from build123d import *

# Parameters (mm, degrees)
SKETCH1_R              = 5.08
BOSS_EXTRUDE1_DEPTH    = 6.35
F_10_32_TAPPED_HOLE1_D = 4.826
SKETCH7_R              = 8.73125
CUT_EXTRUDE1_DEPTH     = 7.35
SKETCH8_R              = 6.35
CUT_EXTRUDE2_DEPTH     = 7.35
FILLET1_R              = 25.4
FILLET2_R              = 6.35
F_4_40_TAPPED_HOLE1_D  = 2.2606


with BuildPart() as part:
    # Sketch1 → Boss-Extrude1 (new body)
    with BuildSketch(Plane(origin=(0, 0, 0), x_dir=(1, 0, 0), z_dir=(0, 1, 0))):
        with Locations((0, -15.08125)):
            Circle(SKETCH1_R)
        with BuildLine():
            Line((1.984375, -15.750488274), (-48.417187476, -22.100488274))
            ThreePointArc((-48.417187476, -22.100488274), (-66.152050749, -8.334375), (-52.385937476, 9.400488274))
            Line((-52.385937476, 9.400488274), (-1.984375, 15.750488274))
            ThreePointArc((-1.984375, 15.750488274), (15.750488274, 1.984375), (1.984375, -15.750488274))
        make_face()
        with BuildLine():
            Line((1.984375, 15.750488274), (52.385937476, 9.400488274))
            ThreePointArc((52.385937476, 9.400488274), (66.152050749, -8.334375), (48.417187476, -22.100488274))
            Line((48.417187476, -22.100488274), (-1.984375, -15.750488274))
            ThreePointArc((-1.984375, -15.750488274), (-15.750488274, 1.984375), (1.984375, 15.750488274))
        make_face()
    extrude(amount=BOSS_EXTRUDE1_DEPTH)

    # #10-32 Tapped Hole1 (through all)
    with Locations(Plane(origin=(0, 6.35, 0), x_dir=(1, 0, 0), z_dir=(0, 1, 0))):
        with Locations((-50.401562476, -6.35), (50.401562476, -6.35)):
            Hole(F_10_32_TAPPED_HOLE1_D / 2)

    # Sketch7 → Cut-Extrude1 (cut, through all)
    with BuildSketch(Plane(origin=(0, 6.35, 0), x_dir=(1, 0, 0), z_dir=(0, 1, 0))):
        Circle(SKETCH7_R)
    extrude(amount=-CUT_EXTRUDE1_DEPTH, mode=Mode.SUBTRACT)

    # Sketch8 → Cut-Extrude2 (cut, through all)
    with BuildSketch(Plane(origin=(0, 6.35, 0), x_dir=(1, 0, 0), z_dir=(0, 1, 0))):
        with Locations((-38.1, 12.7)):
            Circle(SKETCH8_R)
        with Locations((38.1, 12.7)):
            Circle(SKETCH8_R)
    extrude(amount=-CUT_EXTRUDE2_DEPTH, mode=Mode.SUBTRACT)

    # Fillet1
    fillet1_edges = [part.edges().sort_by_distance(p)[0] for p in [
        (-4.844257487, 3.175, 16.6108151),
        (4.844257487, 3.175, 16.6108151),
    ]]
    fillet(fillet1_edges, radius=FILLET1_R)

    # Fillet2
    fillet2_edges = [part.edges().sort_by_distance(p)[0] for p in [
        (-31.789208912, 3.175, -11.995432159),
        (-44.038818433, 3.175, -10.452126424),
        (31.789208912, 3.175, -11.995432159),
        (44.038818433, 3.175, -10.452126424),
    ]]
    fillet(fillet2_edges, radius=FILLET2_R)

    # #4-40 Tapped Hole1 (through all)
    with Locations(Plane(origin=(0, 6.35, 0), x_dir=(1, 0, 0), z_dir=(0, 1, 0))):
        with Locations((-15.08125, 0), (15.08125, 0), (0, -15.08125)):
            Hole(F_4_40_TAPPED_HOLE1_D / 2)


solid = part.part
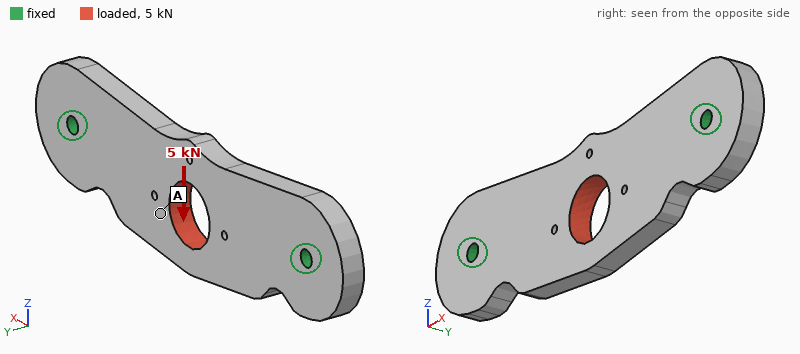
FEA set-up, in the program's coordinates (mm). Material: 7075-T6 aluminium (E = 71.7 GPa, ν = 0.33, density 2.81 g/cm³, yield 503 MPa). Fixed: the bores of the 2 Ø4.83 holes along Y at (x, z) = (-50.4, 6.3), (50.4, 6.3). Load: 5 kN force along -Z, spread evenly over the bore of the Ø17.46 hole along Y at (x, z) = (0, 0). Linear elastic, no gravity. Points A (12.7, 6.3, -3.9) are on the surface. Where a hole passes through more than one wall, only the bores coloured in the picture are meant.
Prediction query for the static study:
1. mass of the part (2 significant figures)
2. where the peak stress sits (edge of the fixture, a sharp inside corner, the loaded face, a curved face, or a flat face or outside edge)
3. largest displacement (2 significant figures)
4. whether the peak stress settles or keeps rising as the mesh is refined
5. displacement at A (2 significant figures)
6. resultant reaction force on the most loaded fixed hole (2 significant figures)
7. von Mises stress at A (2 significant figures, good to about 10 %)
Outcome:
66 g
edge of the fixture
87 µm
keeps rising
76 µm
2.7 kN
33 MPa
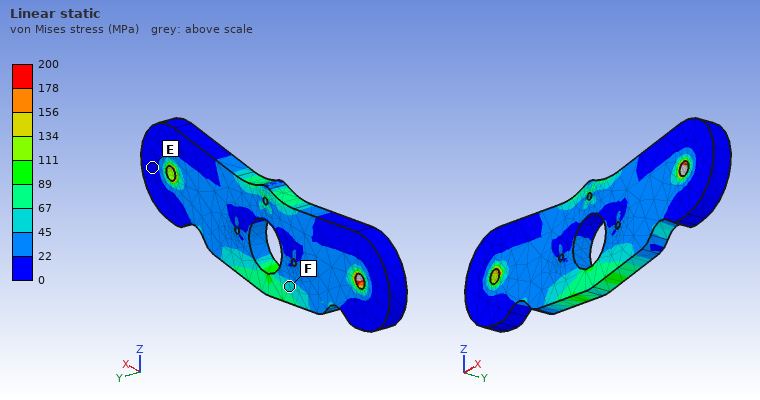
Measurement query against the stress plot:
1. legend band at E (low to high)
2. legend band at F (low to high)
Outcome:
0 to 22 MPa
45 to 67 MPa
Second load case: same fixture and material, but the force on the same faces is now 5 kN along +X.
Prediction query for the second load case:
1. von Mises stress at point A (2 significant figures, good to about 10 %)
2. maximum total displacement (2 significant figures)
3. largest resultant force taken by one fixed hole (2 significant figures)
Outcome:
21 MPa
14 µm
2.5 kN
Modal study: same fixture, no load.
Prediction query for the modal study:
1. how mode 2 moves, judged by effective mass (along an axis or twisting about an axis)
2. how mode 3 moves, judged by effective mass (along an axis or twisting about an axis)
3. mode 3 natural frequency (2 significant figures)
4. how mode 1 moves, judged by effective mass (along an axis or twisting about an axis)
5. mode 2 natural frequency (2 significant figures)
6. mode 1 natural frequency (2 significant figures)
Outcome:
twisting about X
along Z
7600 Hz
along Y
5300 Hz
2900 Hz
